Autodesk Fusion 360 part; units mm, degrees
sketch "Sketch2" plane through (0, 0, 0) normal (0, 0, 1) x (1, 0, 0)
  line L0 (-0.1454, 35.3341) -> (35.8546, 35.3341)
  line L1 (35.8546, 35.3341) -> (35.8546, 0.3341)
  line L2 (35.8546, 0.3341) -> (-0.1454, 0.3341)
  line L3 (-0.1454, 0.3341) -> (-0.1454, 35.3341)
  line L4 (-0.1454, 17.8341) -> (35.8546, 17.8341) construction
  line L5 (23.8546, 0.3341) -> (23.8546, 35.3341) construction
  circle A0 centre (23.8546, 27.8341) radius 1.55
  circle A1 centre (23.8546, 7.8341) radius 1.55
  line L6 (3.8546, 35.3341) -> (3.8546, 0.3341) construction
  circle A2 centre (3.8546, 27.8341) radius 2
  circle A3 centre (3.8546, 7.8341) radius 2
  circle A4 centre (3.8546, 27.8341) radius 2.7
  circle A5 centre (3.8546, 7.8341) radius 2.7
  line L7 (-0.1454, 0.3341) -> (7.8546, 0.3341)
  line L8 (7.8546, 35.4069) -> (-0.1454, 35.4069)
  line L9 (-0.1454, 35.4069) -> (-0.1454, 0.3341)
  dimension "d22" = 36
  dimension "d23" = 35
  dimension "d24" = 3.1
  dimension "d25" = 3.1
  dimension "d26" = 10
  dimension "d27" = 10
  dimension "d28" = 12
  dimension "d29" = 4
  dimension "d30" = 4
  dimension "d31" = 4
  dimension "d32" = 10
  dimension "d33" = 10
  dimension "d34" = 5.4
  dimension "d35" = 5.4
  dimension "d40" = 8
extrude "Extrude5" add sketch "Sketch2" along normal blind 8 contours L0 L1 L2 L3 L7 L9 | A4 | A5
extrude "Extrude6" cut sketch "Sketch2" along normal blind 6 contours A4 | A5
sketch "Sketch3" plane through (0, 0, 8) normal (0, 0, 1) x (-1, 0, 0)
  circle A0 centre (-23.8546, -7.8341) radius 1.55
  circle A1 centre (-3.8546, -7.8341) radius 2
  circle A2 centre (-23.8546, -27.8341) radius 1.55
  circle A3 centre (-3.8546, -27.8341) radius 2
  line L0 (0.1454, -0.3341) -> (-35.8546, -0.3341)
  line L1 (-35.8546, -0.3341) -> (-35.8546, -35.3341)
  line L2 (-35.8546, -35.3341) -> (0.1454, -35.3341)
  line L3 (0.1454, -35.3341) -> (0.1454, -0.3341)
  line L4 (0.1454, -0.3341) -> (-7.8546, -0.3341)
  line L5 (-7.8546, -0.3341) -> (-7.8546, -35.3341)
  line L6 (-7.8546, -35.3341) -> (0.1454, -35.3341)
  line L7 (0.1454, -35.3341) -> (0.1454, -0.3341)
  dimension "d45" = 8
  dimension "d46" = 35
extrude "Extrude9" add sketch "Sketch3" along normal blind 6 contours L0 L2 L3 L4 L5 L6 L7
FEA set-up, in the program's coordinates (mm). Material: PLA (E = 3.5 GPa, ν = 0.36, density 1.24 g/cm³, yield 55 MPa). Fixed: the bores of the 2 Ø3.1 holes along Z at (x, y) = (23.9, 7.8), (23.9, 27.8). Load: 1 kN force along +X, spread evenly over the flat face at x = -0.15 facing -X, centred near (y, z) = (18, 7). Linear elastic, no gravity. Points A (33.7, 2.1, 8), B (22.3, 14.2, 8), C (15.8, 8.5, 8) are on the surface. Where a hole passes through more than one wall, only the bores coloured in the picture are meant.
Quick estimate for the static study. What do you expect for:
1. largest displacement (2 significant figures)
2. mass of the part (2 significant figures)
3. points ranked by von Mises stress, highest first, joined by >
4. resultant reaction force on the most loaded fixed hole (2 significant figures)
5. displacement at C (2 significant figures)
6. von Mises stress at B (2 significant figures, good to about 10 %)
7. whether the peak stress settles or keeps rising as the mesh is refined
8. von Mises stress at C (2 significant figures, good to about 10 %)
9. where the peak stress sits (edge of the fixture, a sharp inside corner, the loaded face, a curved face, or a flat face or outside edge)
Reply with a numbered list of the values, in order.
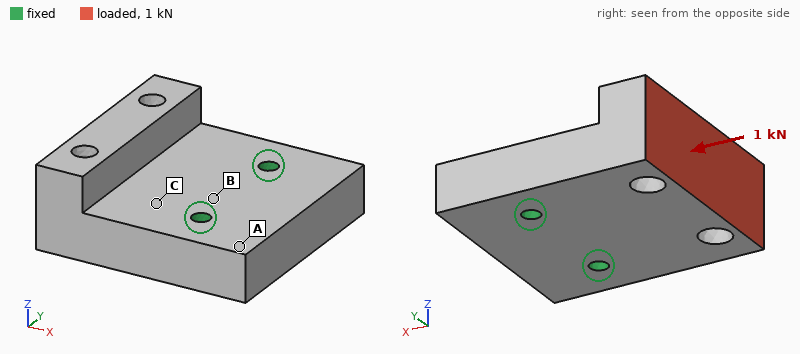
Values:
1. 0.24 mm
2. 14 g
3. C > B > A
4. 500 N
5. 0.044 mm
6. 6.2 MPa
7. keeps rising
8. 12 MPa
9. edge of the fixture
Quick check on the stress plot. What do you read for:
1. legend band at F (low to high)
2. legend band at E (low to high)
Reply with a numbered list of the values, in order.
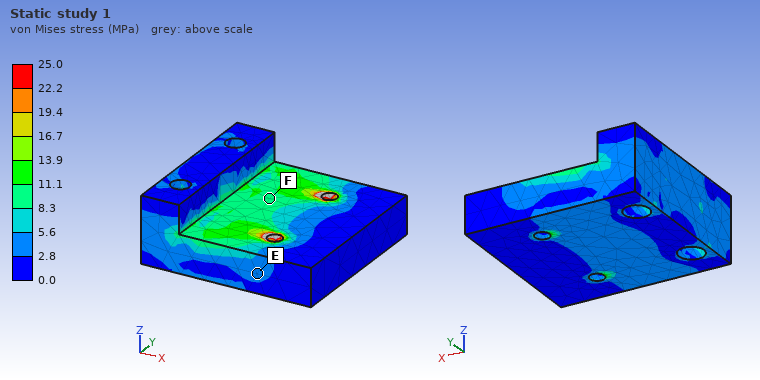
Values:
1. 8.3 to 11.1 MPa
2. 2.8 to 5.6 MPa
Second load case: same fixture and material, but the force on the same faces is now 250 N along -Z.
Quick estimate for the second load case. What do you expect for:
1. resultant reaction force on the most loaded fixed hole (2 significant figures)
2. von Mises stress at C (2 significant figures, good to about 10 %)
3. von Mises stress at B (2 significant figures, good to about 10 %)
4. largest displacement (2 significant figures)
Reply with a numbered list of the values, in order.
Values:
1. 130 N
2. 11 MPa
3. 7.8 MPa
4. 0.32 mm
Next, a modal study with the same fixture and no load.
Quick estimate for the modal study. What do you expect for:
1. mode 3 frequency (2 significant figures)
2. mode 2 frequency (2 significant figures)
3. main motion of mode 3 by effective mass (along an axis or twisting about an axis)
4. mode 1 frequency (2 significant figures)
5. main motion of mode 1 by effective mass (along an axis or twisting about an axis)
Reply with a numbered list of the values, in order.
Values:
1. 6200 Hz
2. 4600 Hz
3. along Y
4. 2500 Hz
5. along Z
